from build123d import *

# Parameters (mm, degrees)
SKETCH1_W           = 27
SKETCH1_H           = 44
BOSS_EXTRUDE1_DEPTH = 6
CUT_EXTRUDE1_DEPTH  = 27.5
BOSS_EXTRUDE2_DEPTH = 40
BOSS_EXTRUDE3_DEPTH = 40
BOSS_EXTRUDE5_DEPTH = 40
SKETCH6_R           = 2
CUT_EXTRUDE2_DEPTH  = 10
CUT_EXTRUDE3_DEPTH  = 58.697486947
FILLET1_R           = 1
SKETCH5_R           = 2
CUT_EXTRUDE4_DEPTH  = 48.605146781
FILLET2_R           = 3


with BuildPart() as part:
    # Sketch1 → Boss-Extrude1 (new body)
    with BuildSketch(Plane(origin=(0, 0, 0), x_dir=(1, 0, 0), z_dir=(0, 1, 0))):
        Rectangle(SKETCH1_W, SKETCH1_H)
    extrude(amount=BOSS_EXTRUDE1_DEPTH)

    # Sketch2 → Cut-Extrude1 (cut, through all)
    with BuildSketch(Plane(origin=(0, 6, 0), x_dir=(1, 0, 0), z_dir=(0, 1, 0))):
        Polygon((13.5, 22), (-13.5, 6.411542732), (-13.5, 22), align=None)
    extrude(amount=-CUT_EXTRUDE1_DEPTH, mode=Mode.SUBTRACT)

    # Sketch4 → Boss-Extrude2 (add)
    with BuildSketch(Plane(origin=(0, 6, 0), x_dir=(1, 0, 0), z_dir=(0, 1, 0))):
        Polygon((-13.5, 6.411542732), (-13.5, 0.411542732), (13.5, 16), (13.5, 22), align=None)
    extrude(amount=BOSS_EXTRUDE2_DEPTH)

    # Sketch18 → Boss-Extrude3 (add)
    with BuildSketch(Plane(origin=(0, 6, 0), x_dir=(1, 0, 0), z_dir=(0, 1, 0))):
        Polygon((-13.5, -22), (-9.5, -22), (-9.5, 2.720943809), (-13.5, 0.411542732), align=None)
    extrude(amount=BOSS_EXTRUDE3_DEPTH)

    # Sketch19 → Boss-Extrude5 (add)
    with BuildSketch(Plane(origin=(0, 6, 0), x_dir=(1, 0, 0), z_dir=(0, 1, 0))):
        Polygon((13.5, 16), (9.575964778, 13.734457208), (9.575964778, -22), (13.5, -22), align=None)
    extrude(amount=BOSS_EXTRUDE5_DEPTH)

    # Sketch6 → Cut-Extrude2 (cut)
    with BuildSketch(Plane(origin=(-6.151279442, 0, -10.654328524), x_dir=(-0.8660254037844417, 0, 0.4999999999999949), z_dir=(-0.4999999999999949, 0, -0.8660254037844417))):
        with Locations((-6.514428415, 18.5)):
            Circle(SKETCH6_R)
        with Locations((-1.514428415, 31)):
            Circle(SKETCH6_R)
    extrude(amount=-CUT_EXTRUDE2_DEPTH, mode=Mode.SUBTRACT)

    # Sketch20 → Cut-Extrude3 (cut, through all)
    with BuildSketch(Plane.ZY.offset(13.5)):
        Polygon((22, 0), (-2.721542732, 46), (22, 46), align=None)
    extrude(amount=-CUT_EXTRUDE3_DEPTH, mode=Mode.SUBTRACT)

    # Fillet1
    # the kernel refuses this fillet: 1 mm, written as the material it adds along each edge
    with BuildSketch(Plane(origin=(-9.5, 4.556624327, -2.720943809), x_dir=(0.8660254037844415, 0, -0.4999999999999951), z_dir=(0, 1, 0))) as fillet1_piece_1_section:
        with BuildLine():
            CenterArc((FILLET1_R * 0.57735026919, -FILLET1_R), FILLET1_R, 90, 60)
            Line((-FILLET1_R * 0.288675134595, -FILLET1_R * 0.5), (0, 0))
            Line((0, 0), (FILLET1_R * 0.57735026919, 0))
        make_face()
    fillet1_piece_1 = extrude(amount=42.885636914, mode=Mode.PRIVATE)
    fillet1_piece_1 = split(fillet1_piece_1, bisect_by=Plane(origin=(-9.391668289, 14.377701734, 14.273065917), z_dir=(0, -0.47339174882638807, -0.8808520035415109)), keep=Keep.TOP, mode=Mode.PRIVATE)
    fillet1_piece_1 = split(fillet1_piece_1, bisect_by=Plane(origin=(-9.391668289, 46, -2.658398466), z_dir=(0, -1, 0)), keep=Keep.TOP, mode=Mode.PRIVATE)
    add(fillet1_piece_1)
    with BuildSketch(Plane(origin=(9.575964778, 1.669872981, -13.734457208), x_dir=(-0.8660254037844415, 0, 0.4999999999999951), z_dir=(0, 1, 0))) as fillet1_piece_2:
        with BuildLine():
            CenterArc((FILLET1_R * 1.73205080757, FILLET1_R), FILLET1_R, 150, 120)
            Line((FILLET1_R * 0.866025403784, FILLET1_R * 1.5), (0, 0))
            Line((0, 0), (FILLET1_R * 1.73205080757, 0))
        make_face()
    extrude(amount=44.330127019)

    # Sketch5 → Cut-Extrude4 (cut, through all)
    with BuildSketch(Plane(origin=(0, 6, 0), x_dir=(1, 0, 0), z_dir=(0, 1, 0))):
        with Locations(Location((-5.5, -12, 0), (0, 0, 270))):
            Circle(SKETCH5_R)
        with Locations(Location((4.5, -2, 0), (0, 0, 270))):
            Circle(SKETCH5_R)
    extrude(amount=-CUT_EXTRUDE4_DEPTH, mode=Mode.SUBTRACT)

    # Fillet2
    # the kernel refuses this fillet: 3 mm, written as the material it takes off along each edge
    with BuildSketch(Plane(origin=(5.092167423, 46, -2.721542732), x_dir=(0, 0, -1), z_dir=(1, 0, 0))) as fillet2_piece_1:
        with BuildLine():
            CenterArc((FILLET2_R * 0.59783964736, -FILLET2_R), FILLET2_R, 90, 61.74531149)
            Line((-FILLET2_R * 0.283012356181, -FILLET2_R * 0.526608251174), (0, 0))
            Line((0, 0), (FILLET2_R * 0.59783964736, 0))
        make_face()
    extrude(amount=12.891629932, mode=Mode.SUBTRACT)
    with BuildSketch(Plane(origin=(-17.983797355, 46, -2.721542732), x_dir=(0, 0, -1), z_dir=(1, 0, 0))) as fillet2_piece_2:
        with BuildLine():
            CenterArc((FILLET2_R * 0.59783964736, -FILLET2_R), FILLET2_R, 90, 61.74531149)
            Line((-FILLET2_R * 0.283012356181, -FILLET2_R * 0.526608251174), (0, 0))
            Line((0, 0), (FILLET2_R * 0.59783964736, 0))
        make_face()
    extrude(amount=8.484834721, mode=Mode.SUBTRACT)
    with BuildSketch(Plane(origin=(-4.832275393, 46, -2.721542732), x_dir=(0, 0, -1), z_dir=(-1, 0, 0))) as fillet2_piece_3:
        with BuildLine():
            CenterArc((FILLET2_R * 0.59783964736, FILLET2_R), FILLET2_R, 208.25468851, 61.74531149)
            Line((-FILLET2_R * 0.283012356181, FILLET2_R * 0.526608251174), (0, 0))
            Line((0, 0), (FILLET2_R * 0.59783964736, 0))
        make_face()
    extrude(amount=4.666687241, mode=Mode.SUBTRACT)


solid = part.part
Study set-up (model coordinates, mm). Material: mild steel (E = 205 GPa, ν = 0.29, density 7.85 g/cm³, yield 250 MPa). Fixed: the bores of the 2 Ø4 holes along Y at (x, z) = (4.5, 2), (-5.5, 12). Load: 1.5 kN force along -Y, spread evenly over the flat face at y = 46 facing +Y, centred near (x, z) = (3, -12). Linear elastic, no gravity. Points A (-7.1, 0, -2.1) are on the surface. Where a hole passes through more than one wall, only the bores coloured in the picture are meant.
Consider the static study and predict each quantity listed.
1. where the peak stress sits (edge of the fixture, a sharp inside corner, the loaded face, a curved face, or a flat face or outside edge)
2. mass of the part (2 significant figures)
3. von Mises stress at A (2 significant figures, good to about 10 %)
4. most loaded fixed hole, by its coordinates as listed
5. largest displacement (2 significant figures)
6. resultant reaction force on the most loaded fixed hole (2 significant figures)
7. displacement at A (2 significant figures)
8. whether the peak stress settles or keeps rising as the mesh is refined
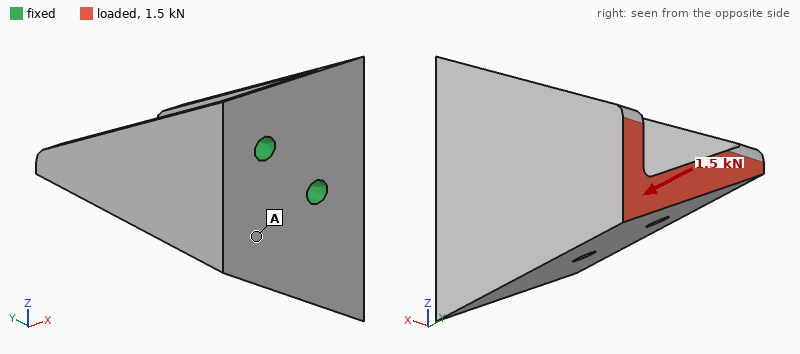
edge of the fixture
130 g
17 MPa
(4.5, 2)
31 µm
1.8 kN
5.4 µm
keeps rising
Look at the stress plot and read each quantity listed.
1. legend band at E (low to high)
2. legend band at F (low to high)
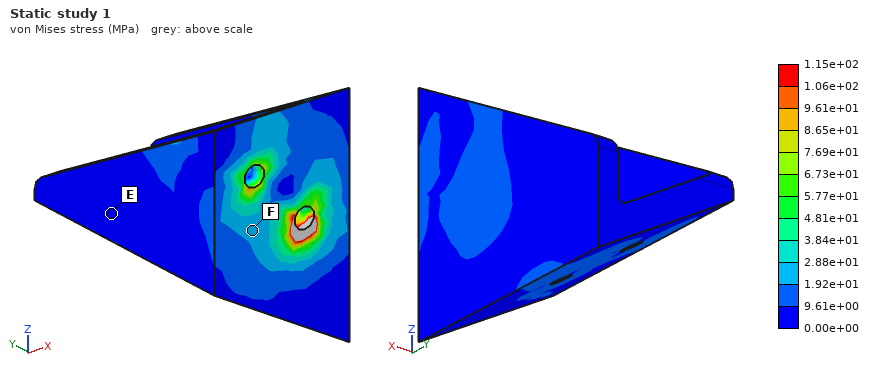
0.00e+00 to 9.61e+00 MPa
1.92e+01 to 2.88e+01 MPa
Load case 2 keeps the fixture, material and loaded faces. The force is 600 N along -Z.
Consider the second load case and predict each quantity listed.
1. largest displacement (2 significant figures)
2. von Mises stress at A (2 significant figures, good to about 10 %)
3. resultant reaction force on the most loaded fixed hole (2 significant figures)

37 µm
16 MPa
850 N
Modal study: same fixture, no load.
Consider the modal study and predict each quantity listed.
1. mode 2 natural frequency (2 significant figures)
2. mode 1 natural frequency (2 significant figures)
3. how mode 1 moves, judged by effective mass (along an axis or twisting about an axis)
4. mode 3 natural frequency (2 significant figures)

4000 Hz
3100 Hz
along X
9600 Hz
